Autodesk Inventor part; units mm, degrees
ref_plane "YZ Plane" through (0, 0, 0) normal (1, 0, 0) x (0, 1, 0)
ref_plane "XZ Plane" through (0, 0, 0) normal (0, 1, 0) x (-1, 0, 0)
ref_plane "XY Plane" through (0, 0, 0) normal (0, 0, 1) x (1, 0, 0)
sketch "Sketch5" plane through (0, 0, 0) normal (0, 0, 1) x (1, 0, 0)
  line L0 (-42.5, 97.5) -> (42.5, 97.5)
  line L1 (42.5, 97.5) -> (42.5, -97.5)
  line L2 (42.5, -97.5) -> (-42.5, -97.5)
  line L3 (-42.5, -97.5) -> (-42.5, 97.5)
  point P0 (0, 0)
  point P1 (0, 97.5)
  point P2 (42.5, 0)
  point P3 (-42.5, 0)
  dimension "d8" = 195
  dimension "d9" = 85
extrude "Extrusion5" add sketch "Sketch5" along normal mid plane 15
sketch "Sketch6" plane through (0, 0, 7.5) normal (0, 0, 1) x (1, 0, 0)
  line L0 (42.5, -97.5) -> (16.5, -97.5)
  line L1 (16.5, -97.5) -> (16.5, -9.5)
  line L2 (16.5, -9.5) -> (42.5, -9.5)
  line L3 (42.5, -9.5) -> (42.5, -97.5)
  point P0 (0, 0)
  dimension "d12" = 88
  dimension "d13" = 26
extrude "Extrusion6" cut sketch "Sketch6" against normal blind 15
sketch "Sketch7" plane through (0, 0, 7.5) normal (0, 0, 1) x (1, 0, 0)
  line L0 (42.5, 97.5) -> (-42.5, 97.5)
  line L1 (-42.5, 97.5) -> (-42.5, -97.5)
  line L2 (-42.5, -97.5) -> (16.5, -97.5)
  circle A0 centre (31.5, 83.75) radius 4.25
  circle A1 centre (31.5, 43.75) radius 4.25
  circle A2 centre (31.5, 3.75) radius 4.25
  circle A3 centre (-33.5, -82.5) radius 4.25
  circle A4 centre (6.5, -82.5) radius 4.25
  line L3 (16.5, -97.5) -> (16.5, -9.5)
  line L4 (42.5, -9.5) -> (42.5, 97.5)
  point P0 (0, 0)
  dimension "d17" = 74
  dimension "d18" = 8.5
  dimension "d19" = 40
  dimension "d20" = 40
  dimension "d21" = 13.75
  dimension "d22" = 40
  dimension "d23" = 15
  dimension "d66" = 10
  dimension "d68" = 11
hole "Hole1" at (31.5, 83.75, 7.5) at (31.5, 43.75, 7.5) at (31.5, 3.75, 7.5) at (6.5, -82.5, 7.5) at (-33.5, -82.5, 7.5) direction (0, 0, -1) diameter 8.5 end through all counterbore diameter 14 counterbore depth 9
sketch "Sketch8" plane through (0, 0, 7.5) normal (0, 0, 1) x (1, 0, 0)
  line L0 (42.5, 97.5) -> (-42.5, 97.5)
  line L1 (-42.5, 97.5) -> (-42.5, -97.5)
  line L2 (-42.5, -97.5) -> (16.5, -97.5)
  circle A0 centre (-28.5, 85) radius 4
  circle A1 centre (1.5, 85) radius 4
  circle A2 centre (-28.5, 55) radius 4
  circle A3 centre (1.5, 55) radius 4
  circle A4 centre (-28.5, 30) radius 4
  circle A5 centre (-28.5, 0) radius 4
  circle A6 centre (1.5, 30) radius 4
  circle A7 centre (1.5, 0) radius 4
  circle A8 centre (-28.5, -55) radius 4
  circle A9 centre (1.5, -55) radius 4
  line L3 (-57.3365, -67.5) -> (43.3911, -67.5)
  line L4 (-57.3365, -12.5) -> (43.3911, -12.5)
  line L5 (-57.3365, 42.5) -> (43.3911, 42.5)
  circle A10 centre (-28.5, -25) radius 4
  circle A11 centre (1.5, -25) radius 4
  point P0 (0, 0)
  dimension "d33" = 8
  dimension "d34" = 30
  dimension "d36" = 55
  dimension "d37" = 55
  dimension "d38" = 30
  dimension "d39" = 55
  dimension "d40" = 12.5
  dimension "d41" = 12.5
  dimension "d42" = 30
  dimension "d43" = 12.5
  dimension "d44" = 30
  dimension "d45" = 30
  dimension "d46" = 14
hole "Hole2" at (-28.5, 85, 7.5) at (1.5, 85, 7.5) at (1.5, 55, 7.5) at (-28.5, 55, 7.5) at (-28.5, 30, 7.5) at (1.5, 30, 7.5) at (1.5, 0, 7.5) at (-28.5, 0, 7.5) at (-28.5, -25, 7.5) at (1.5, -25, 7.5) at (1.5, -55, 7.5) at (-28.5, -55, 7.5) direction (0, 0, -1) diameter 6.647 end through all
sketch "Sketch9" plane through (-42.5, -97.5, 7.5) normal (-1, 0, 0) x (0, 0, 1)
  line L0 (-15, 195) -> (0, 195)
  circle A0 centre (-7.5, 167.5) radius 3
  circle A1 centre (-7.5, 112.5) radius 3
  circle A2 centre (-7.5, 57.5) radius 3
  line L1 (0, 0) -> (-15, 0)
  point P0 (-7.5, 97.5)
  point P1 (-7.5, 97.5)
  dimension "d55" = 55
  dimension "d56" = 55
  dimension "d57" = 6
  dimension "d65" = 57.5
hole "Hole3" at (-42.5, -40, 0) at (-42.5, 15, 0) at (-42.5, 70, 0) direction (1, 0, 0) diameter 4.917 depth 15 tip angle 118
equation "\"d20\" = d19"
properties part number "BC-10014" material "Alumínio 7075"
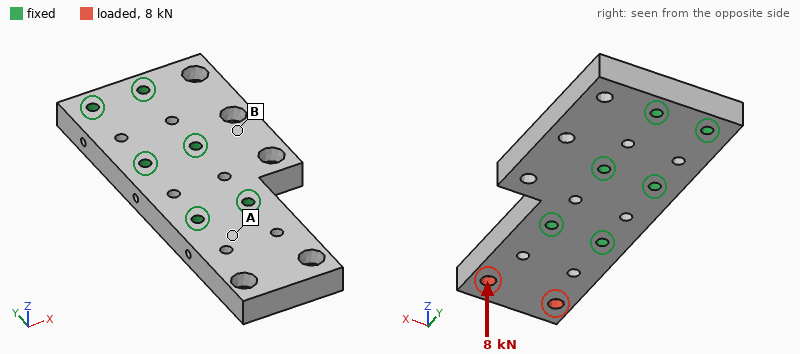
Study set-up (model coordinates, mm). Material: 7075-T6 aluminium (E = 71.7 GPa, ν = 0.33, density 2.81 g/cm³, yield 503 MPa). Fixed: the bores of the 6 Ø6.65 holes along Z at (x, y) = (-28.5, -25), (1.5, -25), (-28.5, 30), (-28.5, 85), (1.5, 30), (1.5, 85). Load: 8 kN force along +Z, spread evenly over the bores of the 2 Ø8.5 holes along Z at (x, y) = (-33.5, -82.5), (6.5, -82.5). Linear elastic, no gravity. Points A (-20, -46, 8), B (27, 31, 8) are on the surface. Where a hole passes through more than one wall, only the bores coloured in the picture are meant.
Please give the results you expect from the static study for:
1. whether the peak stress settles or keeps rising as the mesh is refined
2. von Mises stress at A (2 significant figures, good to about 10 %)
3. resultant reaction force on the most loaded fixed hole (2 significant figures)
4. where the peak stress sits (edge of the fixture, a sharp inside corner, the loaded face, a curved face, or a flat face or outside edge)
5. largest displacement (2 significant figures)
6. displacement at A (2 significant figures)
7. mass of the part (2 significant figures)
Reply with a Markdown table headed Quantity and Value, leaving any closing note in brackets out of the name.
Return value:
| Quantity | Value |
|---|---|
| whether the peak stress settles or keeps rising as the mesh is refined | keeps rising |
| von Mises stress at A | 130 MPa |
| resultant reaction force on the most loaded fixed hole | 5.1 kN |
| where the peak stress sits | edge of the fixture |
| largest displacement | 0.67 mm |
| displacement at A | 0.11 mm |
| mass of the part | 560 g |
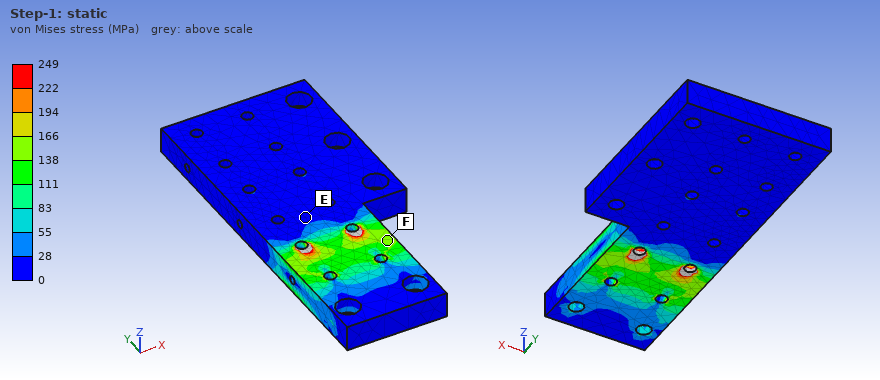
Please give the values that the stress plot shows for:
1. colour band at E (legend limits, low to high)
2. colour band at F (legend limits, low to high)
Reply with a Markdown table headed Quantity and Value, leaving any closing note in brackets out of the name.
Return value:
| Quantity | Value |
|---|---|
| colour band at E | 0 to 28 MPa |
| colour band at F | 138 to 166 MPa |
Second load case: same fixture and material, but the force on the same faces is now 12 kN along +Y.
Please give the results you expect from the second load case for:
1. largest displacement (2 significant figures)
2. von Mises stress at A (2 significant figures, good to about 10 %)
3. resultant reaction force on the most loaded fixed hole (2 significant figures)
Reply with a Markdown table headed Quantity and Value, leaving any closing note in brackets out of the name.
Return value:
| Quantity | Value |
|---|---|
| largest displacement | 0.13 mm |
| von Mises stress at A | 9.7 MPa |
| resultant reaction force on the most loaded fixed hole | 5.6 kN |
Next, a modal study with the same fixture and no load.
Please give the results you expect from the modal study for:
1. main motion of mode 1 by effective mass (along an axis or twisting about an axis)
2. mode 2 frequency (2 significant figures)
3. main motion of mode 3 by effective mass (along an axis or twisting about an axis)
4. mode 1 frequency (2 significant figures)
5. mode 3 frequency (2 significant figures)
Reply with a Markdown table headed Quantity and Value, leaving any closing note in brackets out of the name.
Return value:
| Quantity | Value |
|---|---|
| main motion of mode 1 by effective mass | along Z |
| mode 2 frequency | 5700 Hz |
| main motion of mode 3 by effective mass | along X |
| mode 1 frequency | 2300 Hz |
| mode 3 frequency | 6000 Hz |
